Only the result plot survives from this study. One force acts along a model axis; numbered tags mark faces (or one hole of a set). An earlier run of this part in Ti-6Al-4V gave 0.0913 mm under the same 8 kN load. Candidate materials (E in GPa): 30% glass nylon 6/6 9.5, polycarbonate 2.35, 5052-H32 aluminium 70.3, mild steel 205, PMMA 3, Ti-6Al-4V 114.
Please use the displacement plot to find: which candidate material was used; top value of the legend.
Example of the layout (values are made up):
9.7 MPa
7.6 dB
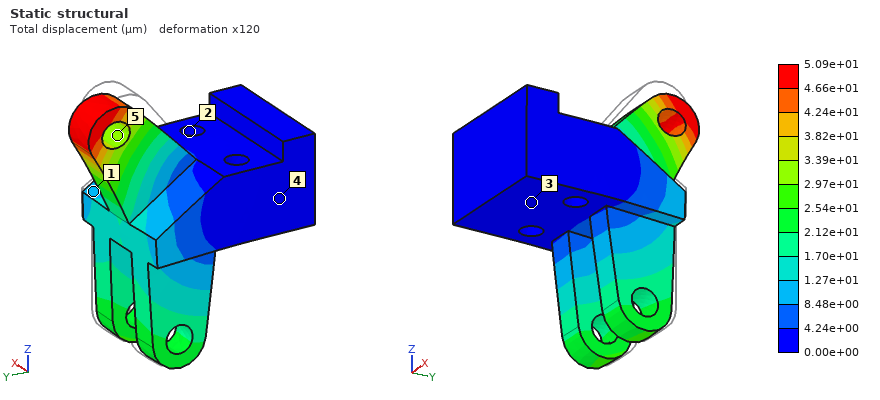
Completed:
mild steel
5.09e+01 µm
